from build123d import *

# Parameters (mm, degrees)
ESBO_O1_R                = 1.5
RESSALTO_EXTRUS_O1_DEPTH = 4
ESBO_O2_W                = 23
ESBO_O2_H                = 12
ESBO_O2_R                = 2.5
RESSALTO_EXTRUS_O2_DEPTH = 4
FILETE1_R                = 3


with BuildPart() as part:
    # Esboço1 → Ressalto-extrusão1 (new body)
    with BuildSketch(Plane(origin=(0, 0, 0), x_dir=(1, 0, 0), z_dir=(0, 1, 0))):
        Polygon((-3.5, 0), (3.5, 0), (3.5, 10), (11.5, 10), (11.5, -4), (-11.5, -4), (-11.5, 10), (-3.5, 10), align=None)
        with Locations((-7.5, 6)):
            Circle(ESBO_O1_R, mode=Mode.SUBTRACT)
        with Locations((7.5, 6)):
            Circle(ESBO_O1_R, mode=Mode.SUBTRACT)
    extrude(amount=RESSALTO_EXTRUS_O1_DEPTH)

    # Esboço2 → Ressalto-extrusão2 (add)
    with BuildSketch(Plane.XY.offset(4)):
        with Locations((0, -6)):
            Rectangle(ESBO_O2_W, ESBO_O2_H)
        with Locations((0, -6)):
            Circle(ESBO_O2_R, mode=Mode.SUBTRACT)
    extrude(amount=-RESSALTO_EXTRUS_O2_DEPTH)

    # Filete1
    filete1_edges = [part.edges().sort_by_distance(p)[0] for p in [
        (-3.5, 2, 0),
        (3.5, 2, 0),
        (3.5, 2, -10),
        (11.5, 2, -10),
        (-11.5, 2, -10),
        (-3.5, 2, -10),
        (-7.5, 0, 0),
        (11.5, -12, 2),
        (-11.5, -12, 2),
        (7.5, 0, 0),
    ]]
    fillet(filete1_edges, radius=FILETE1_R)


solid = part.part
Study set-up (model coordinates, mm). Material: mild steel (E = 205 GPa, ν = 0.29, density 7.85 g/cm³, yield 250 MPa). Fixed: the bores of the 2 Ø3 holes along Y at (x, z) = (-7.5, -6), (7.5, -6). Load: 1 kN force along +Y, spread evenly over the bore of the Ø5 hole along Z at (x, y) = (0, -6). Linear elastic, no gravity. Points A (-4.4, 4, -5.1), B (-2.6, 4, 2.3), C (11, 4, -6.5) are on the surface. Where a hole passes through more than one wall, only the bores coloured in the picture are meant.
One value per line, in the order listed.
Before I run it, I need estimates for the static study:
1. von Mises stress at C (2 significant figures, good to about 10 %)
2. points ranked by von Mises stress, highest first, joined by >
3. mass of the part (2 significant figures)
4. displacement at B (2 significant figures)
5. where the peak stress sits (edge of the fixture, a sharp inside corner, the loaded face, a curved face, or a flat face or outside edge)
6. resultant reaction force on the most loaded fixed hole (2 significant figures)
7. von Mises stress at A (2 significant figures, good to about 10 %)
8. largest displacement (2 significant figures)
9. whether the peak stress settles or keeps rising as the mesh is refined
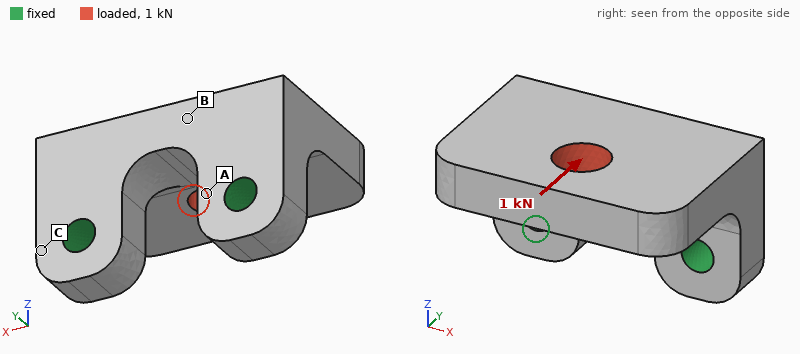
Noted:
43 MPa
A > C > B
16 g
10 µm
edge of the fixture
500 N
82 MPa
25 µm
keeps rising
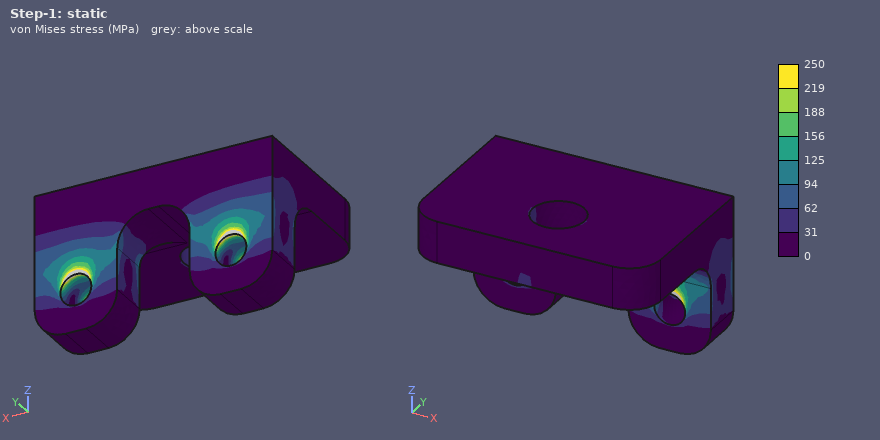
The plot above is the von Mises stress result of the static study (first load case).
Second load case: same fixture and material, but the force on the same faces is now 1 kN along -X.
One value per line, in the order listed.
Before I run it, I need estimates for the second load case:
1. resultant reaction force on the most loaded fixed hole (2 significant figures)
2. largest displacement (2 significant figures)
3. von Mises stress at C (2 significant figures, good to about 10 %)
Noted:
730 N
11 µm
41 MPa
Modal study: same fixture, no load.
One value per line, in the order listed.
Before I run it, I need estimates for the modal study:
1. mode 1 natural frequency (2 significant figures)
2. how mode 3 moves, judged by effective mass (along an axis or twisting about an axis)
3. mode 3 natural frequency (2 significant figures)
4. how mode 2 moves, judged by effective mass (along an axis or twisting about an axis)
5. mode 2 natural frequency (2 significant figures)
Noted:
9100 Hz
along X
26 kHz
along X
17 kHz
